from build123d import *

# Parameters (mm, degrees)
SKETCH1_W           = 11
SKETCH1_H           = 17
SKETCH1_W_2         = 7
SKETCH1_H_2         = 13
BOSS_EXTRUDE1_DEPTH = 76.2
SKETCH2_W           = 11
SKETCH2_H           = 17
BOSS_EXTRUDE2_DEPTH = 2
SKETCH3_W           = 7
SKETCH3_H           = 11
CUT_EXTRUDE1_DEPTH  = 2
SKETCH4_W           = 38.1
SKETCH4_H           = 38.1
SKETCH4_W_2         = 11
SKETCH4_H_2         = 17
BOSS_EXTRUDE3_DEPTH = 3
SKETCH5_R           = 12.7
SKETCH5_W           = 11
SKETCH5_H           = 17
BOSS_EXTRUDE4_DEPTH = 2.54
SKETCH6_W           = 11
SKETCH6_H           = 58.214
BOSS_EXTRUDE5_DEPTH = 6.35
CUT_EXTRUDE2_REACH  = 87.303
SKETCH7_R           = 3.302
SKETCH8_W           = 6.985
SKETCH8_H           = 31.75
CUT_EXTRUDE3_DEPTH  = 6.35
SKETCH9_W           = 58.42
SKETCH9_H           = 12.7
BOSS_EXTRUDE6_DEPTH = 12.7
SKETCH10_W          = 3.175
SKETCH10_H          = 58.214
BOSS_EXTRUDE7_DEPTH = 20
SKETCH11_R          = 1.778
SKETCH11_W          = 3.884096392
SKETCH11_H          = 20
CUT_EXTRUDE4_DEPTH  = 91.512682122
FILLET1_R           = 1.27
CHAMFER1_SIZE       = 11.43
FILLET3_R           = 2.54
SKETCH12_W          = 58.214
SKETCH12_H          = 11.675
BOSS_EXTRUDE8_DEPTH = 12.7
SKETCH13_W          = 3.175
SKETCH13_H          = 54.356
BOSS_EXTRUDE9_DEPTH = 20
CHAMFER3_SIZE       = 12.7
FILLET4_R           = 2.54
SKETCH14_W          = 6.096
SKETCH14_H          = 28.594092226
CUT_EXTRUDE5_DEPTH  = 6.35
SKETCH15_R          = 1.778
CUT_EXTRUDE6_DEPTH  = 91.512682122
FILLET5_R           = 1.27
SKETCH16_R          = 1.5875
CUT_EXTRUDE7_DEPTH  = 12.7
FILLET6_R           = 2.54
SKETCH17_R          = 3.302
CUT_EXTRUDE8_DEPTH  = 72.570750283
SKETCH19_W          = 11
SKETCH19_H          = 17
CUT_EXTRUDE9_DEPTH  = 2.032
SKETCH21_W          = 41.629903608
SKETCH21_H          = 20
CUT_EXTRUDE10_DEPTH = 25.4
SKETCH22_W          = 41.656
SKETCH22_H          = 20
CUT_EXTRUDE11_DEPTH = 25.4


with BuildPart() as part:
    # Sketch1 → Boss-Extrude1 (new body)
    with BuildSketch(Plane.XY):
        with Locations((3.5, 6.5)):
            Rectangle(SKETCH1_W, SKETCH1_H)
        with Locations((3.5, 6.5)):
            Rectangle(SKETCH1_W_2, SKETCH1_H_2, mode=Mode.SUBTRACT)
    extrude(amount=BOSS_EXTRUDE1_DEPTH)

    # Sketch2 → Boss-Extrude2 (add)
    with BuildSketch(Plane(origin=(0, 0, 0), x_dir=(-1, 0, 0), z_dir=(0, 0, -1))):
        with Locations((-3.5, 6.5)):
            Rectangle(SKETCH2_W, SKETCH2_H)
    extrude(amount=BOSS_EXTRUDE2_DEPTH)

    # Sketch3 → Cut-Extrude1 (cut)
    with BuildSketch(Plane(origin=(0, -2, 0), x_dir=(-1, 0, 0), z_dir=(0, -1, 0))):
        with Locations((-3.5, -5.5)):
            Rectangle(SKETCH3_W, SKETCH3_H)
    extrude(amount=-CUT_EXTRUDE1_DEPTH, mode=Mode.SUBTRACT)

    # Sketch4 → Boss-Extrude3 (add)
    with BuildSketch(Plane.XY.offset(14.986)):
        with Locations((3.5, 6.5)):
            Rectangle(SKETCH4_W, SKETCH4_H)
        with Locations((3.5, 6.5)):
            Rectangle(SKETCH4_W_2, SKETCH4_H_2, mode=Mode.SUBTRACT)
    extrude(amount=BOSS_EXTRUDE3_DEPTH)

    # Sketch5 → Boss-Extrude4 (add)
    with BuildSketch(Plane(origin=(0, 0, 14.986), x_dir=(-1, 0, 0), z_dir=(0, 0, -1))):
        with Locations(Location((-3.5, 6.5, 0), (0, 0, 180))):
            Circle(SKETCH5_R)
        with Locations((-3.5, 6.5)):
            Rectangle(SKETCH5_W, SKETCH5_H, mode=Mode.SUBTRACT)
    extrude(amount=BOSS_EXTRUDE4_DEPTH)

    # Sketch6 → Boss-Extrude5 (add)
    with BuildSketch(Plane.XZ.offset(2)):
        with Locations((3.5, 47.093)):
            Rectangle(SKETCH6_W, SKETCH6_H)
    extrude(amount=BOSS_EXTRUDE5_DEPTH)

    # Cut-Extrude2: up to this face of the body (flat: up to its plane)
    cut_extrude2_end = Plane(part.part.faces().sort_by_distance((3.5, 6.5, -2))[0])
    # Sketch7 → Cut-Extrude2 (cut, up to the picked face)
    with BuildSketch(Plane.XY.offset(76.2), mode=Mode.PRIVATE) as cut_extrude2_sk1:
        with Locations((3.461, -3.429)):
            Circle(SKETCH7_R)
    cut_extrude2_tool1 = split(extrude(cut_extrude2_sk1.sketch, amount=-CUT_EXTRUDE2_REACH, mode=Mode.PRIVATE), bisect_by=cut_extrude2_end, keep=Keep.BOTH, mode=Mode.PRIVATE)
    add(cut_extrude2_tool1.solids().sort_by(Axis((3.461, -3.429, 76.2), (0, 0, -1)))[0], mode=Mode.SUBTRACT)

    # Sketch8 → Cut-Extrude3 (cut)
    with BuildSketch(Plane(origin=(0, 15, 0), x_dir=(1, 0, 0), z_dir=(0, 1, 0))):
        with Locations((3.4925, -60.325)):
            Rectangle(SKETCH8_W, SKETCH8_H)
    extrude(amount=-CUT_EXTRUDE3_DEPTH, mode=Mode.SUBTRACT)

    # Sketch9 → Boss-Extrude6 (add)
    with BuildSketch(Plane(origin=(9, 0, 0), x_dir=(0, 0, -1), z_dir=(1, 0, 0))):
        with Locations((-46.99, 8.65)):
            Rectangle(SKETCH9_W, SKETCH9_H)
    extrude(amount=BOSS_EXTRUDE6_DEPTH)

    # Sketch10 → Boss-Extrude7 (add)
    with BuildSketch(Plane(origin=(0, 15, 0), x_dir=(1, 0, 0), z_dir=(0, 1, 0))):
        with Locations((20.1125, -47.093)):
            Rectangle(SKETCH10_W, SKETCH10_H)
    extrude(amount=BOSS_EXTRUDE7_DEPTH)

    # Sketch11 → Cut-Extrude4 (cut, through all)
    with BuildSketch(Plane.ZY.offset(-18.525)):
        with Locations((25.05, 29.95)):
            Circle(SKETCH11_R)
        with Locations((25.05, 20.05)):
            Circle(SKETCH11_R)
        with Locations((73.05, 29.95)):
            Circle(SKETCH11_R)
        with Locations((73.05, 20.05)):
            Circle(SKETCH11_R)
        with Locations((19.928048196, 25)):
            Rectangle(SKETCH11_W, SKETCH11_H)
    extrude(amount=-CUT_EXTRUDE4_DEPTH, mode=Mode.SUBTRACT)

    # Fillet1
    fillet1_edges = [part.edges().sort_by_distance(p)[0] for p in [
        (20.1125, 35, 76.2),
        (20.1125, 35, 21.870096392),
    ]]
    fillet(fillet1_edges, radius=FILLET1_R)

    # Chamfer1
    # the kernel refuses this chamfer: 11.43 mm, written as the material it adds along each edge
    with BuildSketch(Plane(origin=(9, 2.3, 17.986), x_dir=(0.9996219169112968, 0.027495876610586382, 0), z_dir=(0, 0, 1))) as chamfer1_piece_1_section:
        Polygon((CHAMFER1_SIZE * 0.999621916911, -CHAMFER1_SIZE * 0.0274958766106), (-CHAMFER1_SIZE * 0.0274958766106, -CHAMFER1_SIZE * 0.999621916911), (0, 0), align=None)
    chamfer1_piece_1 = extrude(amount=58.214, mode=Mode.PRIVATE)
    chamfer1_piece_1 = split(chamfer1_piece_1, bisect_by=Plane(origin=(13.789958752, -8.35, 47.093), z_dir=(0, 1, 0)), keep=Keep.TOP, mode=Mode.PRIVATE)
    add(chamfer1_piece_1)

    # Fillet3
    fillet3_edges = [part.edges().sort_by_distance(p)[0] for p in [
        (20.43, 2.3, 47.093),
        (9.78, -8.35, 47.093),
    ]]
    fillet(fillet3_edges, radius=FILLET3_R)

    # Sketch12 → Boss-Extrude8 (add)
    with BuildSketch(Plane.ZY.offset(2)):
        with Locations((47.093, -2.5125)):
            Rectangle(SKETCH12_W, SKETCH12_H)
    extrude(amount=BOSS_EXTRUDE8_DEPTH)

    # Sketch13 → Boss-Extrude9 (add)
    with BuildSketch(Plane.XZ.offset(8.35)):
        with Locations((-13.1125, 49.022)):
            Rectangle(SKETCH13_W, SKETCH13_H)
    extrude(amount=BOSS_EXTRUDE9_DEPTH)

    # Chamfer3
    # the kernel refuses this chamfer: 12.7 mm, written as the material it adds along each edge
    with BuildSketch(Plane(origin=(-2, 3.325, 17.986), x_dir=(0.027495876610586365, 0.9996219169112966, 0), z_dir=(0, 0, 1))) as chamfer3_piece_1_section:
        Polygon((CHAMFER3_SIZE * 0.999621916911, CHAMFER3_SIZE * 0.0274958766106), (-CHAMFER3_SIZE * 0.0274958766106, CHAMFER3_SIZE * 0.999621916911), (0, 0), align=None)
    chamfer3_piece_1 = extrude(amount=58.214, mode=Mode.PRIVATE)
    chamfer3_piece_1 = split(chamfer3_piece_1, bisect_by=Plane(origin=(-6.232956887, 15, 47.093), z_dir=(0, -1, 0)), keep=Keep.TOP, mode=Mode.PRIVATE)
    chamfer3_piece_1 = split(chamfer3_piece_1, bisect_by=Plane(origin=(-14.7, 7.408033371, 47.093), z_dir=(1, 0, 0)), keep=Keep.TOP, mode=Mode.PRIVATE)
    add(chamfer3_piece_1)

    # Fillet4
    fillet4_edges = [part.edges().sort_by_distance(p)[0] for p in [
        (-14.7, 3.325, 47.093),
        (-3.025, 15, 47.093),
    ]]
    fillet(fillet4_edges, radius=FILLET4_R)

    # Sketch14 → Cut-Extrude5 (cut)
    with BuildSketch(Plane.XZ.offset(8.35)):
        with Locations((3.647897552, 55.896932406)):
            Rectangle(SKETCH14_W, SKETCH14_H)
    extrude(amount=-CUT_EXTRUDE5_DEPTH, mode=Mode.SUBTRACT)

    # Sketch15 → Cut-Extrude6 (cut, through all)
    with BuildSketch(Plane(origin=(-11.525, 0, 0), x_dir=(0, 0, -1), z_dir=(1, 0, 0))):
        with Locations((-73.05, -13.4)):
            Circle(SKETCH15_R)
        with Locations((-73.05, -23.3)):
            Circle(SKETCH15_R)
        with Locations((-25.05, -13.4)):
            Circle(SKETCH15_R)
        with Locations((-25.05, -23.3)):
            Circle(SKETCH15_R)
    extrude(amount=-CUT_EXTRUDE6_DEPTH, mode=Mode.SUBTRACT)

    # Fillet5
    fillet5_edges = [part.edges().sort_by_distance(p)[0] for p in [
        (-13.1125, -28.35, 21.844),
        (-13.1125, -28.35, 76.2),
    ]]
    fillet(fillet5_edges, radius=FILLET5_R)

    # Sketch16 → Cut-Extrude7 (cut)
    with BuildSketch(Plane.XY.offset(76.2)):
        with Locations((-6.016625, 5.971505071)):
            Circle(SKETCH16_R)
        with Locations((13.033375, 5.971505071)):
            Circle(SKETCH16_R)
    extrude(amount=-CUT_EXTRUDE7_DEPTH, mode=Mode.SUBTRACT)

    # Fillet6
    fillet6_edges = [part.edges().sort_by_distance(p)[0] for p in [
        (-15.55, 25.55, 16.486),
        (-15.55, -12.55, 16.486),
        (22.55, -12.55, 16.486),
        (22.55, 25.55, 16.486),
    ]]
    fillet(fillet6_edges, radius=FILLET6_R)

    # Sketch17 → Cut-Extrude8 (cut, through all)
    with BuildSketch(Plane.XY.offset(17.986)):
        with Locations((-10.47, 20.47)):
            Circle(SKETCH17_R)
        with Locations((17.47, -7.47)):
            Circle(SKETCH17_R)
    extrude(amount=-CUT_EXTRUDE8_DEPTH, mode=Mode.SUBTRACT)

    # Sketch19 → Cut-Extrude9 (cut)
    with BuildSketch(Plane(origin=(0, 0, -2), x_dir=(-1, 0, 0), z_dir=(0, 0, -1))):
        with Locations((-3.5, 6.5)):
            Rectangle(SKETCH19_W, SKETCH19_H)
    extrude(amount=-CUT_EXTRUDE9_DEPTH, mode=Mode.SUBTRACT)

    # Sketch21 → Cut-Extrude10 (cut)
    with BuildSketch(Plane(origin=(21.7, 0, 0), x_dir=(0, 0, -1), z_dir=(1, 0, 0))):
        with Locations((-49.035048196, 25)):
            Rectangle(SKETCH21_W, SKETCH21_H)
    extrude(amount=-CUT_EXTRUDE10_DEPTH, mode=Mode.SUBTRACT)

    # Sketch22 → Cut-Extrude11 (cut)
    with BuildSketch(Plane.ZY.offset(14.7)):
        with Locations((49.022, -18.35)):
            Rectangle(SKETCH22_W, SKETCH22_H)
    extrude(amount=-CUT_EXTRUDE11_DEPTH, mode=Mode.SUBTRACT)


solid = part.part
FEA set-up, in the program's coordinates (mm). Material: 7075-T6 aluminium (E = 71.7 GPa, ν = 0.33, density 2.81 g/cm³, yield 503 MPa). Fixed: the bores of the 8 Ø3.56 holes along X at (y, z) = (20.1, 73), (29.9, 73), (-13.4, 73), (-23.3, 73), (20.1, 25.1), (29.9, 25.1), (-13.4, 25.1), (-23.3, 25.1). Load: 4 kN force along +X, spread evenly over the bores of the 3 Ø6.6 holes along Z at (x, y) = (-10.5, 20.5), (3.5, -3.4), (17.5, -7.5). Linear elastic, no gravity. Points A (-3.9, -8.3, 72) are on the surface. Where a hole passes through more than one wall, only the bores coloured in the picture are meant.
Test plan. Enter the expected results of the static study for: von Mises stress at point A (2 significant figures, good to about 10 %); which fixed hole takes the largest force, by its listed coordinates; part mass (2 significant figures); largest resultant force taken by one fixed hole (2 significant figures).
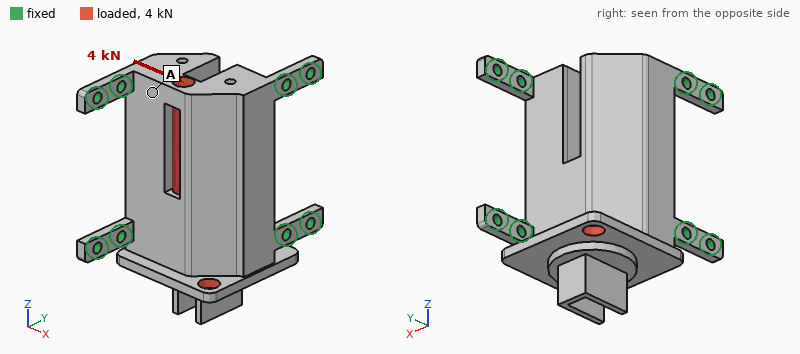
23 MPa
(-13.4, 25.1)
110 g
1.5 kN
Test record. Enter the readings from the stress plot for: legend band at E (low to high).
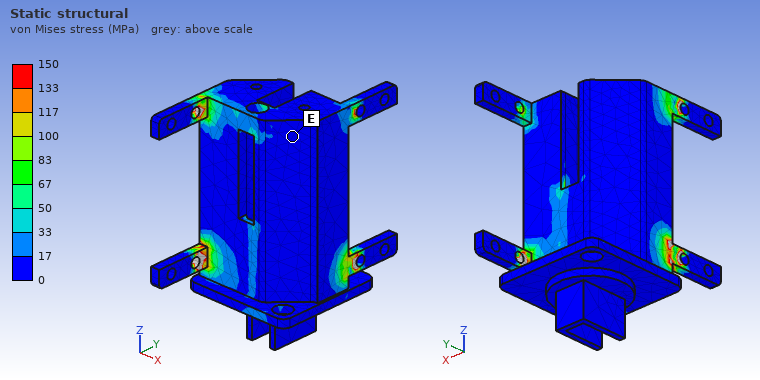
0 to 17 MPa
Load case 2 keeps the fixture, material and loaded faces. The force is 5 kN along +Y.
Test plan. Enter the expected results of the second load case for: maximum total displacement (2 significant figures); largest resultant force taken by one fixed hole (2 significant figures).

35 µm
1.7 kN
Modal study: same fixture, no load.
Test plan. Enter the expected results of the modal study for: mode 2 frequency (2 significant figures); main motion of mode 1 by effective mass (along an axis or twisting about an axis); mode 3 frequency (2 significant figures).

7000 Hz
along X
7100 Hz
